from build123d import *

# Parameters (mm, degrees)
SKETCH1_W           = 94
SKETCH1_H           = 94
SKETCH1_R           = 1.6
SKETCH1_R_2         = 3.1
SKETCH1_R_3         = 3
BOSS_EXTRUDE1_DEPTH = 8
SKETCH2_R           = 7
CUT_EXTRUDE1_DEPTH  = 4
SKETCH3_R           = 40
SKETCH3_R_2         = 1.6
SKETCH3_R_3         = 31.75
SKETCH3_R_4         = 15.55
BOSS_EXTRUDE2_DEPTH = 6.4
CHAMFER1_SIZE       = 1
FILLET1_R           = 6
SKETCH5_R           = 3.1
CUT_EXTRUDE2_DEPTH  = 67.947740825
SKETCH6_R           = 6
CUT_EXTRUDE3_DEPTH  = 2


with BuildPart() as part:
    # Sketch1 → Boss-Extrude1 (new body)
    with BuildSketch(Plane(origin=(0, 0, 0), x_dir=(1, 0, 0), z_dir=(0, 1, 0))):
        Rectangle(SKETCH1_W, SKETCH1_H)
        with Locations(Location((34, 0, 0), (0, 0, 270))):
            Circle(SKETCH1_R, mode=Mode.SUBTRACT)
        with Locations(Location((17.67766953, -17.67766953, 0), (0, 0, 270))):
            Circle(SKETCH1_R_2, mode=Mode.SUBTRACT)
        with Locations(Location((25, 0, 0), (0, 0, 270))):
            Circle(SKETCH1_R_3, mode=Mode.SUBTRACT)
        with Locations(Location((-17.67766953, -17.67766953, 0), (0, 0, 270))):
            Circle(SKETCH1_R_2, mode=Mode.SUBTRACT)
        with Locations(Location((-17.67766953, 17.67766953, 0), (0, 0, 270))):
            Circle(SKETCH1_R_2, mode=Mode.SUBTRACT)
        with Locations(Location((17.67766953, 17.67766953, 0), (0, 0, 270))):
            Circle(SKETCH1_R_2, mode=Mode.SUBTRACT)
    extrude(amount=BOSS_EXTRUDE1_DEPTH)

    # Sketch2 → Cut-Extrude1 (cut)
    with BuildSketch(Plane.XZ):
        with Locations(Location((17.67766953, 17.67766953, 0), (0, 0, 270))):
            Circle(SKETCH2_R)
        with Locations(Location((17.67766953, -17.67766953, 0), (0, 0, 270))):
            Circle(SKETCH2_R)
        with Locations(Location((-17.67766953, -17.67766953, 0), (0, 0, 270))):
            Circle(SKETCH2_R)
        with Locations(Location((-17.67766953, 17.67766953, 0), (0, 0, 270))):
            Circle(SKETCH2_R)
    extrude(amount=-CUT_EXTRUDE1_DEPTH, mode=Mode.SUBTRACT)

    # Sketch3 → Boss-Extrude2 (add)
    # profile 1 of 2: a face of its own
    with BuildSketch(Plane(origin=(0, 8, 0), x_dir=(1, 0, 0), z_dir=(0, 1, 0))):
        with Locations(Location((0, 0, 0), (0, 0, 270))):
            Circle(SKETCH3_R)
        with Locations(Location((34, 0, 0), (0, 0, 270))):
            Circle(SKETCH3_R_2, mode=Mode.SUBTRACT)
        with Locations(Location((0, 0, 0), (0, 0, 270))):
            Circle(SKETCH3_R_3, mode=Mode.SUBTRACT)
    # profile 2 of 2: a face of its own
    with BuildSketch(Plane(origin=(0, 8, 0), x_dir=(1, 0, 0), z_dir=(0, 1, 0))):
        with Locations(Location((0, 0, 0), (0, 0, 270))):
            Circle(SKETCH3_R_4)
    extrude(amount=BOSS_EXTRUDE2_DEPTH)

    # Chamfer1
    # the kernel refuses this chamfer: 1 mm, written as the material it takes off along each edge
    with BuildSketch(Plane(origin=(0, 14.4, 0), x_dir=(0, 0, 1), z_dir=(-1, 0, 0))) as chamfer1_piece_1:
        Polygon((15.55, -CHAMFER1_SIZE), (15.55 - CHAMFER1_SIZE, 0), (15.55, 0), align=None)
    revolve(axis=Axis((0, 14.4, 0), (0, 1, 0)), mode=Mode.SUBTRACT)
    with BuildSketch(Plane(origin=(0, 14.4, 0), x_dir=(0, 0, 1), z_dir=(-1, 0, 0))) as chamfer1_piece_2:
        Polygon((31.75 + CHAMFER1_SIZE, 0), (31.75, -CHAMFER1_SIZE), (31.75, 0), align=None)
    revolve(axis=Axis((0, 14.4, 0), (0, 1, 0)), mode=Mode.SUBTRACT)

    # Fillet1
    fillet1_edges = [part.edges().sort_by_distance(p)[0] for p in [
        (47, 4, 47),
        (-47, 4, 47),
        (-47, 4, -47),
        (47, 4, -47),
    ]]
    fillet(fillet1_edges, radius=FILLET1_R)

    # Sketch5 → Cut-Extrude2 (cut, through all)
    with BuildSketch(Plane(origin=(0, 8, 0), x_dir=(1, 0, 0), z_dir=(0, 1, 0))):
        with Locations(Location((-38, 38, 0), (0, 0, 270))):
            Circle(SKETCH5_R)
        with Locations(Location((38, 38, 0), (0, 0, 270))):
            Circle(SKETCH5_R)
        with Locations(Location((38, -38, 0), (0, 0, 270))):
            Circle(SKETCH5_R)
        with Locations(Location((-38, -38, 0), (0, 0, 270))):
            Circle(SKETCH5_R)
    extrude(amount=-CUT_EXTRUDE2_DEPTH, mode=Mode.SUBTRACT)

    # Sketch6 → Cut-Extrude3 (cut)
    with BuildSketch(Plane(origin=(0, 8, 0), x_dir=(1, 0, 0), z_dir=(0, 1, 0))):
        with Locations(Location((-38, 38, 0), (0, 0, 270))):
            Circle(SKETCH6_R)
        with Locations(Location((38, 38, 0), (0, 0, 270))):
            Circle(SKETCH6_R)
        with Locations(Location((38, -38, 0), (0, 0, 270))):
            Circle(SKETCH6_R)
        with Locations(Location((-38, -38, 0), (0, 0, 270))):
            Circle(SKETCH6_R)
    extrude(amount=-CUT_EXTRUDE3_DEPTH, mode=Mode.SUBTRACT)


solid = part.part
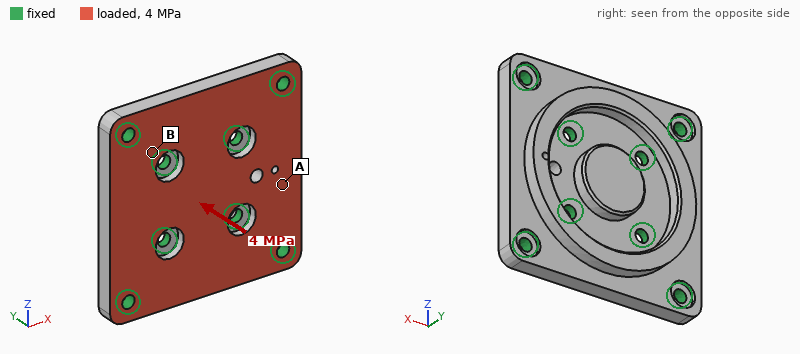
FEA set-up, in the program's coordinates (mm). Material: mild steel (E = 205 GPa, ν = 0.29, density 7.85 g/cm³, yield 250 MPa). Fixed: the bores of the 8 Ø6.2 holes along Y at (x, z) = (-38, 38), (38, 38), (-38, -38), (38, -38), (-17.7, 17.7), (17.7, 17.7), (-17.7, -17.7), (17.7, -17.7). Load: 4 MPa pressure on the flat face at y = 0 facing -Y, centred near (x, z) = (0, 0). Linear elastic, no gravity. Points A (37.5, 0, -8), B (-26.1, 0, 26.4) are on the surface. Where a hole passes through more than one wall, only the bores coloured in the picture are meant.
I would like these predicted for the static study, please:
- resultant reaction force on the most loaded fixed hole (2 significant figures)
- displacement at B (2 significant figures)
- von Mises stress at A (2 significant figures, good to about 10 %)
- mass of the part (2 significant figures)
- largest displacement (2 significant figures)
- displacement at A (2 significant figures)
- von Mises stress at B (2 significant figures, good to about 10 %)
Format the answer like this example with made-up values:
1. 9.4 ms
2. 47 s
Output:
1. 4.7 kN
2. 5.0 µm
3. 17 MPa
4. 640 g
5. 17 µm
6. 11 µm
7. 52 MPa
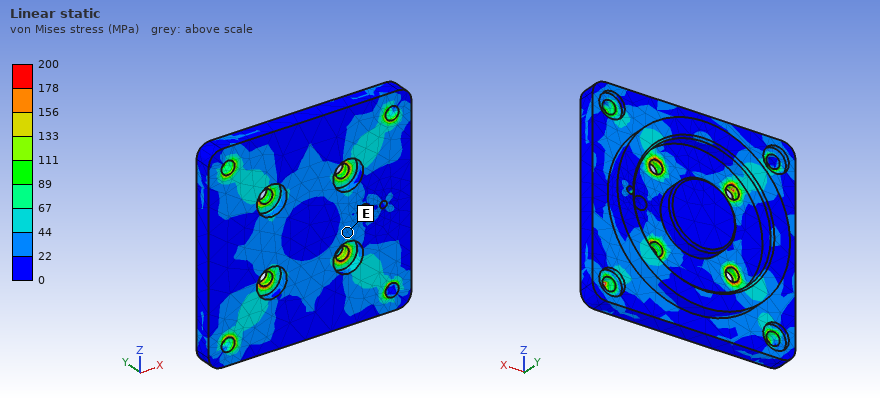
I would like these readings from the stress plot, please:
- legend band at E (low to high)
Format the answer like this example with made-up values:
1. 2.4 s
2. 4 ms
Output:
1. 22 to 44 MPa
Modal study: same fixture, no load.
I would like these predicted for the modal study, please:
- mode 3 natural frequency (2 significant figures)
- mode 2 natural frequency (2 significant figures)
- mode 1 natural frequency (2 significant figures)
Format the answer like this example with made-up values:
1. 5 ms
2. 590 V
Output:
1. 10 kHz
2. 10 kHz
3. 8700 Hz
